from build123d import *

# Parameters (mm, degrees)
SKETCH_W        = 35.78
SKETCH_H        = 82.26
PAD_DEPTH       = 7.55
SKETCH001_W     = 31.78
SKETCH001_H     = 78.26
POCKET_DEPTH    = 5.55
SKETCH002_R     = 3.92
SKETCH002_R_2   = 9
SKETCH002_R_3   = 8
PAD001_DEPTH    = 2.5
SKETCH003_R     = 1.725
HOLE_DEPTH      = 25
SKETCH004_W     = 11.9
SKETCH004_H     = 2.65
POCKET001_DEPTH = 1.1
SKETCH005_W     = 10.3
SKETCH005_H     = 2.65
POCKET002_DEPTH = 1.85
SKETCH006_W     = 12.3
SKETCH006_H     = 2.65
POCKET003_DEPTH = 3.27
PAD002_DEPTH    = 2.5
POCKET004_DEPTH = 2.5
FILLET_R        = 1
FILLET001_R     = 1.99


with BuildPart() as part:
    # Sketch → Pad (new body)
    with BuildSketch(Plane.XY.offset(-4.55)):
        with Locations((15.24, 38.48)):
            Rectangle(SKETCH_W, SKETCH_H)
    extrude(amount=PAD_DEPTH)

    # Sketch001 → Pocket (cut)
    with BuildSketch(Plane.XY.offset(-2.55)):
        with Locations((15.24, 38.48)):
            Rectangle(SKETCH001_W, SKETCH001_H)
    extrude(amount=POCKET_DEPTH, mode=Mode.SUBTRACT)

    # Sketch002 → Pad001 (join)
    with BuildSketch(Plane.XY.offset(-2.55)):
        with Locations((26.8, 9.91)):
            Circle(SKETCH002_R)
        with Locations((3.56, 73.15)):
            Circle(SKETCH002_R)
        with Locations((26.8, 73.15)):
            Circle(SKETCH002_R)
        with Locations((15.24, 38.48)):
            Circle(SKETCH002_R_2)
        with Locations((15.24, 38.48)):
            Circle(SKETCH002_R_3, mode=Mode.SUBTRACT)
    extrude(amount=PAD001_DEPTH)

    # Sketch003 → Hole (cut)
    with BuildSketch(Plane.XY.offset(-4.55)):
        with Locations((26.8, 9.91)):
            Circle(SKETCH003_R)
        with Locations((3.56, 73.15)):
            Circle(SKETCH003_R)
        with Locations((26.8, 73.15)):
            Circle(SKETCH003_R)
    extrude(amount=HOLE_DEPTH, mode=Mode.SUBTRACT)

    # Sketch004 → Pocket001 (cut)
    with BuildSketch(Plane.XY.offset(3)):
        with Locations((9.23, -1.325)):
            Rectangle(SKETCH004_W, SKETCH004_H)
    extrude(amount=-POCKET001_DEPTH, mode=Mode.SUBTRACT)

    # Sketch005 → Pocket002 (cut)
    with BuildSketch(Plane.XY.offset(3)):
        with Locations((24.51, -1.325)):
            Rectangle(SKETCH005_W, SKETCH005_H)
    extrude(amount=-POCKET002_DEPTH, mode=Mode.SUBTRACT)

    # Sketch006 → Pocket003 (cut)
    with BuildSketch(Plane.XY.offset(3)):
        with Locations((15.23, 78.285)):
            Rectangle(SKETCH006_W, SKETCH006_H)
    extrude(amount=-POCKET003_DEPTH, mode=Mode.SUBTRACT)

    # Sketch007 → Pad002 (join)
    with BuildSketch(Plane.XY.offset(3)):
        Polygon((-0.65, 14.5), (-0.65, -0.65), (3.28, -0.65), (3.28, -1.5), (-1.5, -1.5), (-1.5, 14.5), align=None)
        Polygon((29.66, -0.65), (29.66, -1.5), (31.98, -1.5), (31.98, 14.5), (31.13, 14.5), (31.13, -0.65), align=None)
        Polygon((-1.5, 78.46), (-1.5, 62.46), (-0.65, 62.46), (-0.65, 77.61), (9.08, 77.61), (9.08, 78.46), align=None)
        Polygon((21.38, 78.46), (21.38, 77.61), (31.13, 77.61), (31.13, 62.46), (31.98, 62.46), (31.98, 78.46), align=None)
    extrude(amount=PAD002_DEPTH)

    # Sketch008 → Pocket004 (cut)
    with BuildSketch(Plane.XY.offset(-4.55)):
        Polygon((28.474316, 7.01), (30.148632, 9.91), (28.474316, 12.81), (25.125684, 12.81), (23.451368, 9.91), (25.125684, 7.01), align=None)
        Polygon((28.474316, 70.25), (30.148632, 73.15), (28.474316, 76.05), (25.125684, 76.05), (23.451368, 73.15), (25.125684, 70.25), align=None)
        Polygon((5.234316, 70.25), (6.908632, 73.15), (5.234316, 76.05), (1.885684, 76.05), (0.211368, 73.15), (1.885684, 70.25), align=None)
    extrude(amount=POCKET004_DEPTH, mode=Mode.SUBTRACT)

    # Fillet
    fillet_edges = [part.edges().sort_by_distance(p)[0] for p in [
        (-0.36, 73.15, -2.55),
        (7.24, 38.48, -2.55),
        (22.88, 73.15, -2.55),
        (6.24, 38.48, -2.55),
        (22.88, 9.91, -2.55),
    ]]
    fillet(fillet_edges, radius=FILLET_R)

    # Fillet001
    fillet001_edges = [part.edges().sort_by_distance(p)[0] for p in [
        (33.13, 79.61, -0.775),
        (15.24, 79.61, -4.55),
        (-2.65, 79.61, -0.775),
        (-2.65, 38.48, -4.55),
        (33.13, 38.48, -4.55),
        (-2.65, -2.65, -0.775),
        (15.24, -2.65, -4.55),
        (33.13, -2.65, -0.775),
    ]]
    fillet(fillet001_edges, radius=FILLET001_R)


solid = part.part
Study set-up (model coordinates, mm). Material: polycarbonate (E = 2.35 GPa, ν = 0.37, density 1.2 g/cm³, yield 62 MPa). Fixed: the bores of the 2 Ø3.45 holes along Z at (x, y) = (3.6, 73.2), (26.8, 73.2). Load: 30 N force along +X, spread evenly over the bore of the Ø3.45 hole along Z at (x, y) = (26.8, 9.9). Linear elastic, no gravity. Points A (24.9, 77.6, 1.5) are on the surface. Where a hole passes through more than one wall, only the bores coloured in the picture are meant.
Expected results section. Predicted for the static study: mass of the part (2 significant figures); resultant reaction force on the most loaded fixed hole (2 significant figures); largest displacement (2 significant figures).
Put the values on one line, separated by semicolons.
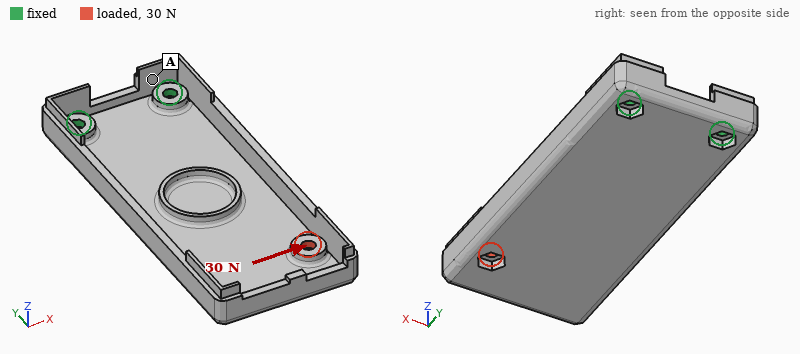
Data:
10 g; 73 N; 1.0 mm
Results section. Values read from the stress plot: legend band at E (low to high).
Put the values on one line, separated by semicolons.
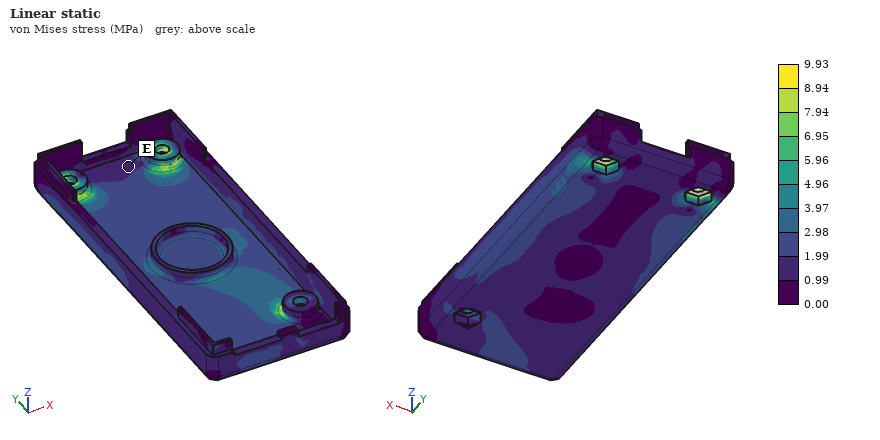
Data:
0.99 to 1.99 MPa
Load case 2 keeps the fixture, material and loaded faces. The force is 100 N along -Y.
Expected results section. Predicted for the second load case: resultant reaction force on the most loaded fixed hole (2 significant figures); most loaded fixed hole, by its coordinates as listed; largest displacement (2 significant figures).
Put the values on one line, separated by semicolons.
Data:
95 N; (26.8, 73.2); 0.92 mm
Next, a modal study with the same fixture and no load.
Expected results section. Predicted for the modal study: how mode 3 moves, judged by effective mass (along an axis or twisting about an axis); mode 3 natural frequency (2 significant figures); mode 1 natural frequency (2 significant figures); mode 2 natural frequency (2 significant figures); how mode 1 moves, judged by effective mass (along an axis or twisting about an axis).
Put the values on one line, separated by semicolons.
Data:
along X; 920 Hz; 160 Hz; 350 Hz; along Z
